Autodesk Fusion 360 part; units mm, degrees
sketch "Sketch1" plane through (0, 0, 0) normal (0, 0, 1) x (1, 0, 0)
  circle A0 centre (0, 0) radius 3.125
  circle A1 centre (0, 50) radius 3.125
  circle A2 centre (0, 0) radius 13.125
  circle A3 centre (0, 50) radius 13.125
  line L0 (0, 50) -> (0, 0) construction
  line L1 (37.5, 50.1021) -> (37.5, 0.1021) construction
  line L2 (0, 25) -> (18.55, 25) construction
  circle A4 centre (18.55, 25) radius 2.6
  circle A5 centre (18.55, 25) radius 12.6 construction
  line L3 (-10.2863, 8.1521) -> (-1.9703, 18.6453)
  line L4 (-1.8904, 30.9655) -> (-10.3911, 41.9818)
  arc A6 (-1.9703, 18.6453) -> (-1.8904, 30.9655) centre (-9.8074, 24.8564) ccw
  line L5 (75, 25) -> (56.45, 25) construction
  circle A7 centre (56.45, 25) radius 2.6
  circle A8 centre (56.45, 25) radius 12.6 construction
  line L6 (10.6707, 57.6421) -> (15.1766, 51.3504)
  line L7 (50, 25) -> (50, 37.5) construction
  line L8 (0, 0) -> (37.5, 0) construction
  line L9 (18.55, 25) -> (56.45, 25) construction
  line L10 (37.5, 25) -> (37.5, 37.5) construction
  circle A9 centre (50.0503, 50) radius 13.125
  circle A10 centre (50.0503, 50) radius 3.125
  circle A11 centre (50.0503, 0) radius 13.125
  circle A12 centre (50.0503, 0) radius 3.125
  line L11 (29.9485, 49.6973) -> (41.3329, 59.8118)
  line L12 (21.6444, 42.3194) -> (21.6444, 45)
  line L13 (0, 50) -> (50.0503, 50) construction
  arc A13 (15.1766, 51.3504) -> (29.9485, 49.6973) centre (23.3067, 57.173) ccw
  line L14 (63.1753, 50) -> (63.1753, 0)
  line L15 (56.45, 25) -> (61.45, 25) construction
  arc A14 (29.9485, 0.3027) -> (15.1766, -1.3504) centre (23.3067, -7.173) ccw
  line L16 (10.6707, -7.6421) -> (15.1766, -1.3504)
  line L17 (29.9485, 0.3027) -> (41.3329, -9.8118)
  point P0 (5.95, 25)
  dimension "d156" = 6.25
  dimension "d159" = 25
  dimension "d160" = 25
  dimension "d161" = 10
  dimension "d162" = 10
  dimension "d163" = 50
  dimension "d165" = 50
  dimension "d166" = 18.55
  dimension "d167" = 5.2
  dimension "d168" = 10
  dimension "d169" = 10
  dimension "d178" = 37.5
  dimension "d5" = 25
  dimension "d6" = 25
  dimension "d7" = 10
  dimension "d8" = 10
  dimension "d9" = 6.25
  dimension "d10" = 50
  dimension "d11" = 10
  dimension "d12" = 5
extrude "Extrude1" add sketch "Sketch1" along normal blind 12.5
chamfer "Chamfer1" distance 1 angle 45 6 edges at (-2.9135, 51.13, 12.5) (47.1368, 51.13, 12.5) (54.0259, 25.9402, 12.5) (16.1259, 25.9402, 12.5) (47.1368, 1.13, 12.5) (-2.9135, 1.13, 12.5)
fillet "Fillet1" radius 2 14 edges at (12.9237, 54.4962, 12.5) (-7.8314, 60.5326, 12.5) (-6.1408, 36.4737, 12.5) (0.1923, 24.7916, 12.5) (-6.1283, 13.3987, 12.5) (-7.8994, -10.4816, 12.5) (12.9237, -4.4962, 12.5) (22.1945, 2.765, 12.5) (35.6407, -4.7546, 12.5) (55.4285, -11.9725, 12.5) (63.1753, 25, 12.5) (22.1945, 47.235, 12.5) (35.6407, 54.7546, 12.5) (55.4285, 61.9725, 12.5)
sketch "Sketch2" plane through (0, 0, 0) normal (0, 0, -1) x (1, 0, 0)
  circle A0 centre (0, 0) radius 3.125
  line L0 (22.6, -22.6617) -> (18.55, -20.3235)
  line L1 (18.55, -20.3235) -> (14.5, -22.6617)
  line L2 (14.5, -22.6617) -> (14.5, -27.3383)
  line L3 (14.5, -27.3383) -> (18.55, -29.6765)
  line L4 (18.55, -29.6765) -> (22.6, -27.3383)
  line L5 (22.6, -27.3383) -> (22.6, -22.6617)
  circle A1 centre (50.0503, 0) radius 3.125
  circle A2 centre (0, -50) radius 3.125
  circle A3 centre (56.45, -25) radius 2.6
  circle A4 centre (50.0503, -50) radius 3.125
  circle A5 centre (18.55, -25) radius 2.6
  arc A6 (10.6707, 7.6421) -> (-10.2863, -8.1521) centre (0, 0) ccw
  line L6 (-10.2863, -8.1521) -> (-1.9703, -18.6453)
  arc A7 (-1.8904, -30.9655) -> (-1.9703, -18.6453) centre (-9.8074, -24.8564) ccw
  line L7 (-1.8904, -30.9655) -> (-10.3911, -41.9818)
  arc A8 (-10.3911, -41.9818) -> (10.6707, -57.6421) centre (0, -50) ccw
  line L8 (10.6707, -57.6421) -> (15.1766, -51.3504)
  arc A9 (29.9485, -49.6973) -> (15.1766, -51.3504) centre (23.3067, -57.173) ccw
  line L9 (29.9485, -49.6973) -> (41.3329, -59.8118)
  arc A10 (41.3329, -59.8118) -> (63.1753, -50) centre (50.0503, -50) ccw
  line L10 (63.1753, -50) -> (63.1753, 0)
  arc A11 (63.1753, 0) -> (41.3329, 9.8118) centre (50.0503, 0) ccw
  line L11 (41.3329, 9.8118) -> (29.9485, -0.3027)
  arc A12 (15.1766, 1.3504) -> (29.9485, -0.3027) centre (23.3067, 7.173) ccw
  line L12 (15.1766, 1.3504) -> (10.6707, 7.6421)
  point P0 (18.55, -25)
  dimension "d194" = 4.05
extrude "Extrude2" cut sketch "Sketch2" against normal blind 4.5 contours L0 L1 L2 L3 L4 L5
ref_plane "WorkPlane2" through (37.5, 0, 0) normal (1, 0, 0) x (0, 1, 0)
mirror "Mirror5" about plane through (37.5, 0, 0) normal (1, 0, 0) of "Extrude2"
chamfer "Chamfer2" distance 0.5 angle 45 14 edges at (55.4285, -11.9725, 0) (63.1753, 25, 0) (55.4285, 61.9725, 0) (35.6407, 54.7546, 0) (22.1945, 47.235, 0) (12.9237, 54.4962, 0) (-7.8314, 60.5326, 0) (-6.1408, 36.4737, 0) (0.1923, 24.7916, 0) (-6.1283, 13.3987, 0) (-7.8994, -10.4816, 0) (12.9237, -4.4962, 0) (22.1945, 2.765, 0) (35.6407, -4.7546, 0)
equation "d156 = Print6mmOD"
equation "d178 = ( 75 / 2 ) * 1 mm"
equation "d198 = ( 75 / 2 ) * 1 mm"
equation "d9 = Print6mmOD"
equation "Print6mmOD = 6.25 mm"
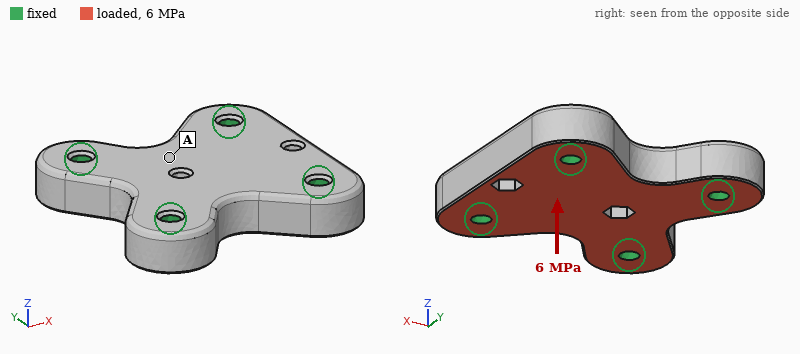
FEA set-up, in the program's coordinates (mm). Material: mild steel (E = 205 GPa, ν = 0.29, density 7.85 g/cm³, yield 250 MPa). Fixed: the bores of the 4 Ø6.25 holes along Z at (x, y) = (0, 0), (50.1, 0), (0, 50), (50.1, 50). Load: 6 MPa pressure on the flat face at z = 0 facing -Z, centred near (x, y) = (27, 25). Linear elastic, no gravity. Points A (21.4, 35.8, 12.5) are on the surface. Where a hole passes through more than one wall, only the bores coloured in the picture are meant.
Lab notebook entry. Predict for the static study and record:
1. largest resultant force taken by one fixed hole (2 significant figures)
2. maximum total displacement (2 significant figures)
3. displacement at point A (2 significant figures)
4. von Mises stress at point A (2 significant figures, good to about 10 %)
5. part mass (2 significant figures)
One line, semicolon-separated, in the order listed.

6.8 kN; 10 µm; 8.8 µm; 26 MPa; 430 g
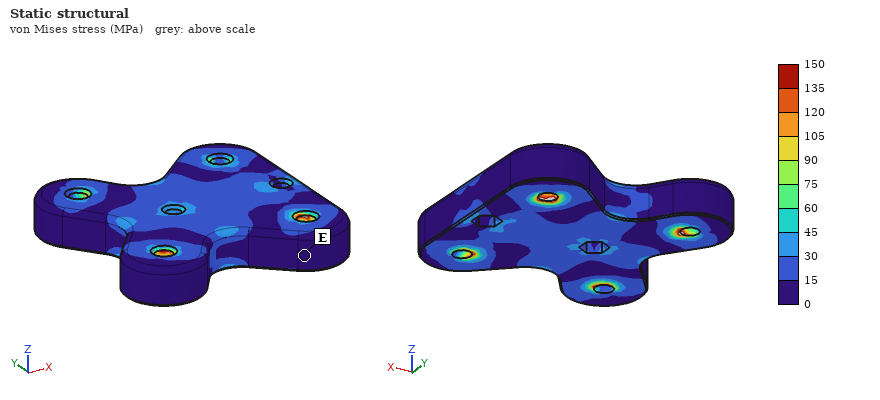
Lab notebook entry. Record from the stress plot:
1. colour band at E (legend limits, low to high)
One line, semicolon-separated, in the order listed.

0 to 15 MPa
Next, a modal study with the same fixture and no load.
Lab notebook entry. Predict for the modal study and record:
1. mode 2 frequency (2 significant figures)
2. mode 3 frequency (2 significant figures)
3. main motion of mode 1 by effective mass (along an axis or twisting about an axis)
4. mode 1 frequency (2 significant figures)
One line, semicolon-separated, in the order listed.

20 kHz; 25 kHz; along Z; 14 kHz
